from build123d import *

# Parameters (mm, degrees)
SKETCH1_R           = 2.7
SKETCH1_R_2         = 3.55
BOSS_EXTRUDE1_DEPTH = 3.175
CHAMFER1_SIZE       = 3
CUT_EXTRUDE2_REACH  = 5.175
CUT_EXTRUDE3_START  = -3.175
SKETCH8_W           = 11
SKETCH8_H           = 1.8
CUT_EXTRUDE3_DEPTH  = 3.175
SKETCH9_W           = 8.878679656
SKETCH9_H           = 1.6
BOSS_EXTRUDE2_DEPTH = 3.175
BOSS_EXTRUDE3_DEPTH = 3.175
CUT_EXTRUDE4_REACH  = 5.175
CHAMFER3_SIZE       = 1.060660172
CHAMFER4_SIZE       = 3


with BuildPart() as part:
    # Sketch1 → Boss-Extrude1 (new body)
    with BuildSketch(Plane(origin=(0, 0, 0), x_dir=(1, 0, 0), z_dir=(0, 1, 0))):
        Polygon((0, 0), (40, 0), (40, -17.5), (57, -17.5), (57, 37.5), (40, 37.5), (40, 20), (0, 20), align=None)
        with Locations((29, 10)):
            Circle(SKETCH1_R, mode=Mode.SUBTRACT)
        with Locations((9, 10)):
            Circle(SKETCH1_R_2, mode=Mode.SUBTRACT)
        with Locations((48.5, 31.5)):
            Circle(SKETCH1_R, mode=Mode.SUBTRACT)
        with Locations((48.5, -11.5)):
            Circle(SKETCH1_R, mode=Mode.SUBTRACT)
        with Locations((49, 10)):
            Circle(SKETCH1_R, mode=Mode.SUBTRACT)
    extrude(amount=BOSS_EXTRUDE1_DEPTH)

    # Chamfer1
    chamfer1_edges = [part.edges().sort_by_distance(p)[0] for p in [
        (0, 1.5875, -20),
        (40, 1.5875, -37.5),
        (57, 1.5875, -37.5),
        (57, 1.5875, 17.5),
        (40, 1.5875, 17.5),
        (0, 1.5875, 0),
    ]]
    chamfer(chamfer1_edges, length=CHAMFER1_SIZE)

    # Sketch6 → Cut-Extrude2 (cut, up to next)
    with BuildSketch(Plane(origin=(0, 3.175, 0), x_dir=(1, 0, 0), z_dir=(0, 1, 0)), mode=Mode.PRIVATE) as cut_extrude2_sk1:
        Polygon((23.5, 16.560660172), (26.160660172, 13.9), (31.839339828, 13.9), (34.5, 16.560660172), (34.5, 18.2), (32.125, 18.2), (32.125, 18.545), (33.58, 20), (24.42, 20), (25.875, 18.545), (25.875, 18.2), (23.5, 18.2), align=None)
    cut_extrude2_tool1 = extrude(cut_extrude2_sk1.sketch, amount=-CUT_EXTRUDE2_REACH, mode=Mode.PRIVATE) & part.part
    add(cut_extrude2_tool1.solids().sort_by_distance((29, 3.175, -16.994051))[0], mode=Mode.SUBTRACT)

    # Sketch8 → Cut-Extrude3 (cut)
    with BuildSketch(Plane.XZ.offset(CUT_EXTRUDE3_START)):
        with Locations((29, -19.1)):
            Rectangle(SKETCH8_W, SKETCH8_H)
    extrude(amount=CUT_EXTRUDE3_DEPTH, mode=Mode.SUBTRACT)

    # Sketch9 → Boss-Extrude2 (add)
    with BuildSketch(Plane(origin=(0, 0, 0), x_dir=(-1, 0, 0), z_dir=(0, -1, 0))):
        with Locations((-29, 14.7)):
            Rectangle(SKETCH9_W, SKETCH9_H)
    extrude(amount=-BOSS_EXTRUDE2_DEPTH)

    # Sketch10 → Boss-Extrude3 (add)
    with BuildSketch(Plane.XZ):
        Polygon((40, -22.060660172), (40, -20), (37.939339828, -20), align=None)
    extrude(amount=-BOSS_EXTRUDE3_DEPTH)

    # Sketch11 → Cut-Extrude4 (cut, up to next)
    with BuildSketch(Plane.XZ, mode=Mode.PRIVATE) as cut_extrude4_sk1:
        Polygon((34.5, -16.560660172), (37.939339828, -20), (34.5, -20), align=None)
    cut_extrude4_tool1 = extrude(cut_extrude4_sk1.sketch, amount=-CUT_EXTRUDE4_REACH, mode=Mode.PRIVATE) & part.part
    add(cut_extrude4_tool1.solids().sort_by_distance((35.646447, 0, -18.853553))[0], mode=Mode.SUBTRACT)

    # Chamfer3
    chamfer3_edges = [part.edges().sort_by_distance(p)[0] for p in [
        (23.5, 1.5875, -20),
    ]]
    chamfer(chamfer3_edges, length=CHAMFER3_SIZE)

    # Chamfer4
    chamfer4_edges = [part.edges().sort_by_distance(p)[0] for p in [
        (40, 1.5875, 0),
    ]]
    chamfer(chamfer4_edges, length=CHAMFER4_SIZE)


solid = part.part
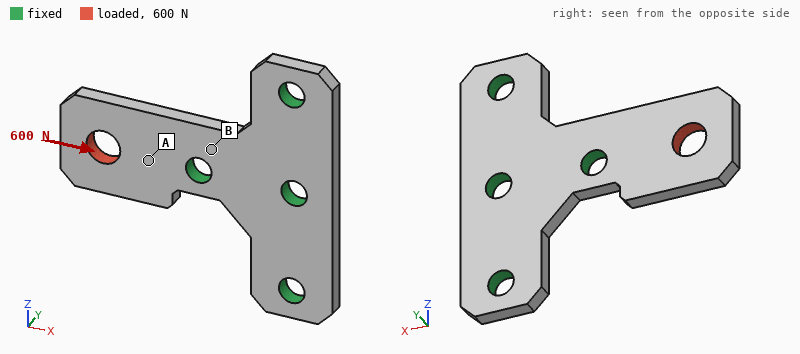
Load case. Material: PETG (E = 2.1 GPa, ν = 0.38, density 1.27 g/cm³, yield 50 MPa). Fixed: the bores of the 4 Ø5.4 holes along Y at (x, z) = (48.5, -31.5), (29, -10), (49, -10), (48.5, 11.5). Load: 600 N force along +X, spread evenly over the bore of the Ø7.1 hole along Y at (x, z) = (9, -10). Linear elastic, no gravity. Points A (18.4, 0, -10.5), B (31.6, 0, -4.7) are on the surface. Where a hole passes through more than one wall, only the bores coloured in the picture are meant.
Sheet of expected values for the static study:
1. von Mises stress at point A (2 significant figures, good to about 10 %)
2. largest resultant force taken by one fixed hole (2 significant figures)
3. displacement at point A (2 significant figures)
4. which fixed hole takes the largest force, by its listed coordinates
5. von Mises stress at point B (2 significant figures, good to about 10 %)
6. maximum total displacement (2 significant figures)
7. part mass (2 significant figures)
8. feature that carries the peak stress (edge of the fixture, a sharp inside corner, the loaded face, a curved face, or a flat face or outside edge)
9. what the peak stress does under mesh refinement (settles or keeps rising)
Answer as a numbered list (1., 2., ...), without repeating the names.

1. 14 MPa
2. 550 N
3. 0.071 mm
4. (29, -10)
5. 3.0 MPa
6. 0.21 mm
7. 6.2 g
8. a sharp inside corner
9. keeps rising
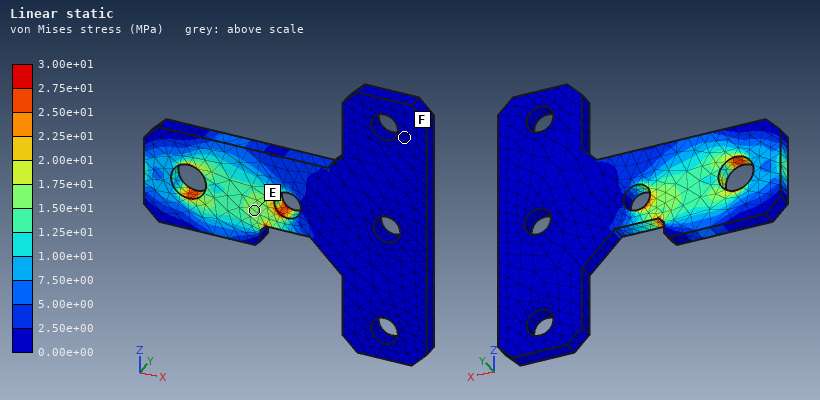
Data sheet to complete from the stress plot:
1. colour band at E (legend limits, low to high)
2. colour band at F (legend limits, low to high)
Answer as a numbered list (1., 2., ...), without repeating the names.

1. 1.50e+01 to 1.75e+01 MPa
2. 0.00e+00 to 2.50e+00 MPa
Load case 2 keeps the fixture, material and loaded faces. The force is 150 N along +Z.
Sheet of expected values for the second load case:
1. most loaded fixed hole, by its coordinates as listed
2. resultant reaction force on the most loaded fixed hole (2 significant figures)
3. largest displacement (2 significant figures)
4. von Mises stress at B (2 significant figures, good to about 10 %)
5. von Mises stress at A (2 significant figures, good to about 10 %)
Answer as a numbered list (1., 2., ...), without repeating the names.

1. (29, -10)
2. 220 N
3. 0.56 mm
4. 7.2 MPa
5. 8.8 MPa
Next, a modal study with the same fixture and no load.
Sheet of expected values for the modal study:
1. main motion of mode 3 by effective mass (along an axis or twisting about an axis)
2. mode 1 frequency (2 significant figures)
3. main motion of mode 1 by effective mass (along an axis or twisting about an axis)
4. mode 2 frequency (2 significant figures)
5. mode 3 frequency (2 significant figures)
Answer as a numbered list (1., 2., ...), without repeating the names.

1. along Z
2. 870 Hz
3. along Y
4. 2100 Hz
5. 2600 Hz
